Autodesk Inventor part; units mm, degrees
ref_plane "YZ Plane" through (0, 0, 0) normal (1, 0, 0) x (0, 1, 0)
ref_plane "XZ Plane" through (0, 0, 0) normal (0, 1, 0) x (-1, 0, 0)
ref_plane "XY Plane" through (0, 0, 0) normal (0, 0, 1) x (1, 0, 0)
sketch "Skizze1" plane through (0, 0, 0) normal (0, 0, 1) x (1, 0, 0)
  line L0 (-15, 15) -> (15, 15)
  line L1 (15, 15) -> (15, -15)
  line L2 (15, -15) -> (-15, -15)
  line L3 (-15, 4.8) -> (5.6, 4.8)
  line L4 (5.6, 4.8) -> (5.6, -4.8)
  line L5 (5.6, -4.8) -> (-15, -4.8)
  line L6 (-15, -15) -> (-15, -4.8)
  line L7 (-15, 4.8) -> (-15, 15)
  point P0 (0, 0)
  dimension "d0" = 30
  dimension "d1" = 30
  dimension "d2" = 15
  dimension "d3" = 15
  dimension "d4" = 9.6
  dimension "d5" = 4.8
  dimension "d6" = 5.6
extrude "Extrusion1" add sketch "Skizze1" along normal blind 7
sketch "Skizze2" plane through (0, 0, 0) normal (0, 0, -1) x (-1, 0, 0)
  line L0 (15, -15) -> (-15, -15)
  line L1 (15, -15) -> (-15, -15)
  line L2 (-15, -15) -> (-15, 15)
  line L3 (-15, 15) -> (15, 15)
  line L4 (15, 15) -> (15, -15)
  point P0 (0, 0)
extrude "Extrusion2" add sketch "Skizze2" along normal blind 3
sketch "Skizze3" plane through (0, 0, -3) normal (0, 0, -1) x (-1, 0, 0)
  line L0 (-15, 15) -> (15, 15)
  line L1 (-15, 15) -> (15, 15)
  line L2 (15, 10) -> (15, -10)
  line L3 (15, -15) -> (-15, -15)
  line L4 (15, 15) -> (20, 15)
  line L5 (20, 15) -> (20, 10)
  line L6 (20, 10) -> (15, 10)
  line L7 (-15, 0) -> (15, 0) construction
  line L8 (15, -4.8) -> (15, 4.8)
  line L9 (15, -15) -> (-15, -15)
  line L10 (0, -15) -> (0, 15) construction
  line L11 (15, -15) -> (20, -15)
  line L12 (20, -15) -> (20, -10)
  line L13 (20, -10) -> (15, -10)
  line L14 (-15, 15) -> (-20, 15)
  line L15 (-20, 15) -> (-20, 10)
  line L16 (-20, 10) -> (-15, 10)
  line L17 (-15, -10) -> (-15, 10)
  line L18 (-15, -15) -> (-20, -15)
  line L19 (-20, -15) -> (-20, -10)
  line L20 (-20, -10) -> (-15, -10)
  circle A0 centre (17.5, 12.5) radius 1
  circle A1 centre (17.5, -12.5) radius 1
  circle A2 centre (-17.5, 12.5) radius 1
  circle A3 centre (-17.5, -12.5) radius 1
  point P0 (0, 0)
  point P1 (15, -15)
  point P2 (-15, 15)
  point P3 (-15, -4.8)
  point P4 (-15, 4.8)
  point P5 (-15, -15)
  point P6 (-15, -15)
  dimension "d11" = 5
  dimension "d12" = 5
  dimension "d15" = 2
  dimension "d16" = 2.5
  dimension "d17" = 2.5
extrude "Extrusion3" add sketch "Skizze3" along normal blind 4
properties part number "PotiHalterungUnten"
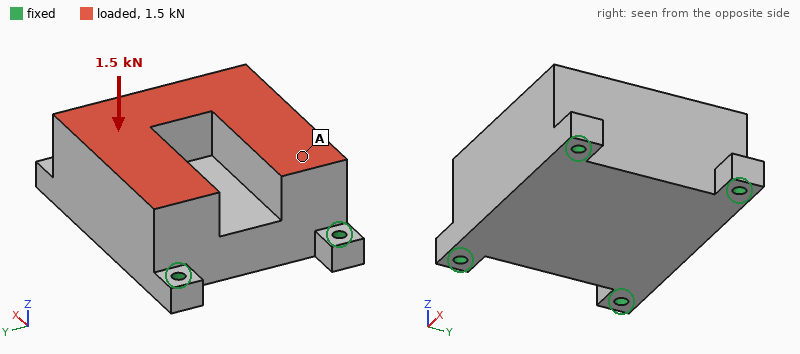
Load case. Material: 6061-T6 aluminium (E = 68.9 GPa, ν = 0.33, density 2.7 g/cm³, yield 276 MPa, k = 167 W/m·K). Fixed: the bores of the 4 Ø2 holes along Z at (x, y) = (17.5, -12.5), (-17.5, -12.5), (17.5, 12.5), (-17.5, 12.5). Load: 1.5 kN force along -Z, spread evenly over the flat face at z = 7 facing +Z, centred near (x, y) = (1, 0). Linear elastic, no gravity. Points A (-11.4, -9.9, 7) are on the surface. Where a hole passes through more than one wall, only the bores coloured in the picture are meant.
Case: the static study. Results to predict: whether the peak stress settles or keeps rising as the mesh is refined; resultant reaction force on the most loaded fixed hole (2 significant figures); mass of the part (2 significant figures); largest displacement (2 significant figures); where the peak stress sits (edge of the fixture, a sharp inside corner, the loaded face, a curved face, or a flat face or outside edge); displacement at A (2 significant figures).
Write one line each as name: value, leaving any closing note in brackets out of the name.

whether the peak stress settles or keeps rising as the mesh is refined: keeps rising
resultant reaction force on the most loaded fixed hole: 450 N
mass of the part: 31 g
largest displacement: 6.1 µm
where the peak stress sits: edge of the fixture
displacement at A: 4.8 µm
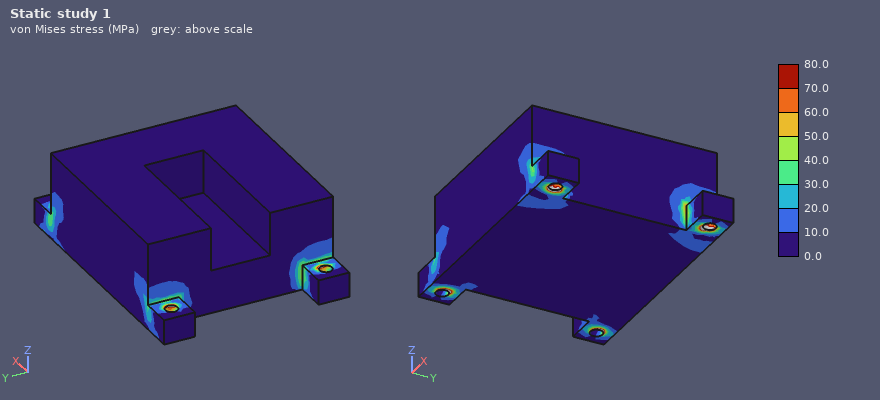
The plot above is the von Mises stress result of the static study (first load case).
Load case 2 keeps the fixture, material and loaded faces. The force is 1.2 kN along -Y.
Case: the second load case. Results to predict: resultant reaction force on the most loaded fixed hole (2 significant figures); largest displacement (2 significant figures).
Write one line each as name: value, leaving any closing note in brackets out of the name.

resultant reaction force on the most loaded fixed hole: 510 N
largest displacement: 10 µm
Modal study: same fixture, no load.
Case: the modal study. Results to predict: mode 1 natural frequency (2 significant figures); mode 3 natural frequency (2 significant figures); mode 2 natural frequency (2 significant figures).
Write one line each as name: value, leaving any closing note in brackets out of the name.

mode 1 natural frequency: 15 kHz
mode 3 natural frequency: 21 kHz
mode 2 natural frequency: 15 kHz
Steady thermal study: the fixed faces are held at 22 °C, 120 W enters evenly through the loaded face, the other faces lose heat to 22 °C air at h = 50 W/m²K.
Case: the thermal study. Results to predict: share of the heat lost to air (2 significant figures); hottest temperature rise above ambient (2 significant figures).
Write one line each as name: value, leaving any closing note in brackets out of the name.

share of the heat lost to air: 5.2 %
hottest temperature rise above ambient: 51 K
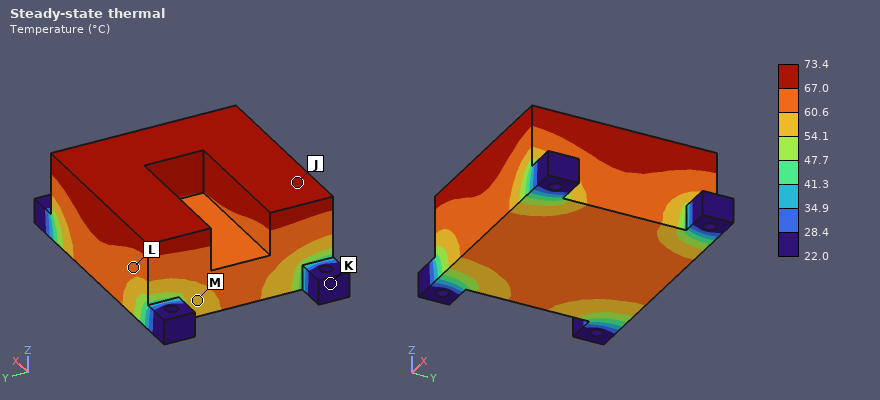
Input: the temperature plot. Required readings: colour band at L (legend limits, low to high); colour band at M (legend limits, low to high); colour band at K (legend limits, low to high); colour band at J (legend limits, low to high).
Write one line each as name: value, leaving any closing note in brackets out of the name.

colour band at L: 60.6 to 67.0 °C
colour band at M: 54.1 to 60.6 °C
colour band at K: 22.0 to 28.4 °C
colour band at J: 67.0 to 73.4 °C
